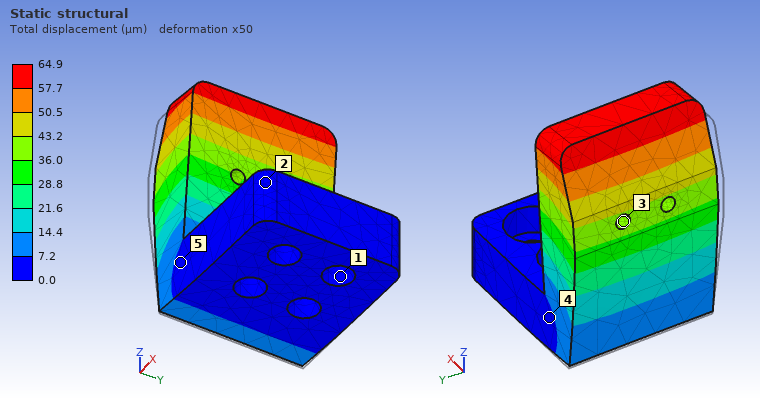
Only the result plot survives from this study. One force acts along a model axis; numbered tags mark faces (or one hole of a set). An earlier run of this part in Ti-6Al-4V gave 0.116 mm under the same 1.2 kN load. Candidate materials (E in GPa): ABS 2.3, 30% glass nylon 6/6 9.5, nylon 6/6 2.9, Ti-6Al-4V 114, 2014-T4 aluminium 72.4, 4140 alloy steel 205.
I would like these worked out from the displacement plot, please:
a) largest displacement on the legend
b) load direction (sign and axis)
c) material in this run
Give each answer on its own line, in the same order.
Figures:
64.9 µm
+X
4140 alloy steel
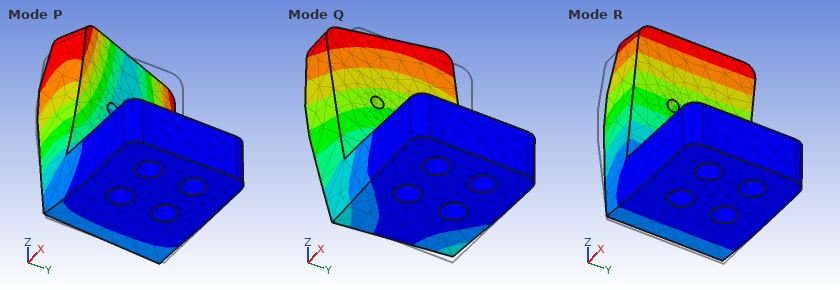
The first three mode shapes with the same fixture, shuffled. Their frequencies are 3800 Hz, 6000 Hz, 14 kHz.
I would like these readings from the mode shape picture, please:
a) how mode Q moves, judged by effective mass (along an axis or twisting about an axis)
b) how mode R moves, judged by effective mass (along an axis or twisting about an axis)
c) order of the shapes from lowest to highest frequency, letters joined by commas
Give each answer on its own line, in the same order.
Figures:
along Y
along X
R, Q, P
